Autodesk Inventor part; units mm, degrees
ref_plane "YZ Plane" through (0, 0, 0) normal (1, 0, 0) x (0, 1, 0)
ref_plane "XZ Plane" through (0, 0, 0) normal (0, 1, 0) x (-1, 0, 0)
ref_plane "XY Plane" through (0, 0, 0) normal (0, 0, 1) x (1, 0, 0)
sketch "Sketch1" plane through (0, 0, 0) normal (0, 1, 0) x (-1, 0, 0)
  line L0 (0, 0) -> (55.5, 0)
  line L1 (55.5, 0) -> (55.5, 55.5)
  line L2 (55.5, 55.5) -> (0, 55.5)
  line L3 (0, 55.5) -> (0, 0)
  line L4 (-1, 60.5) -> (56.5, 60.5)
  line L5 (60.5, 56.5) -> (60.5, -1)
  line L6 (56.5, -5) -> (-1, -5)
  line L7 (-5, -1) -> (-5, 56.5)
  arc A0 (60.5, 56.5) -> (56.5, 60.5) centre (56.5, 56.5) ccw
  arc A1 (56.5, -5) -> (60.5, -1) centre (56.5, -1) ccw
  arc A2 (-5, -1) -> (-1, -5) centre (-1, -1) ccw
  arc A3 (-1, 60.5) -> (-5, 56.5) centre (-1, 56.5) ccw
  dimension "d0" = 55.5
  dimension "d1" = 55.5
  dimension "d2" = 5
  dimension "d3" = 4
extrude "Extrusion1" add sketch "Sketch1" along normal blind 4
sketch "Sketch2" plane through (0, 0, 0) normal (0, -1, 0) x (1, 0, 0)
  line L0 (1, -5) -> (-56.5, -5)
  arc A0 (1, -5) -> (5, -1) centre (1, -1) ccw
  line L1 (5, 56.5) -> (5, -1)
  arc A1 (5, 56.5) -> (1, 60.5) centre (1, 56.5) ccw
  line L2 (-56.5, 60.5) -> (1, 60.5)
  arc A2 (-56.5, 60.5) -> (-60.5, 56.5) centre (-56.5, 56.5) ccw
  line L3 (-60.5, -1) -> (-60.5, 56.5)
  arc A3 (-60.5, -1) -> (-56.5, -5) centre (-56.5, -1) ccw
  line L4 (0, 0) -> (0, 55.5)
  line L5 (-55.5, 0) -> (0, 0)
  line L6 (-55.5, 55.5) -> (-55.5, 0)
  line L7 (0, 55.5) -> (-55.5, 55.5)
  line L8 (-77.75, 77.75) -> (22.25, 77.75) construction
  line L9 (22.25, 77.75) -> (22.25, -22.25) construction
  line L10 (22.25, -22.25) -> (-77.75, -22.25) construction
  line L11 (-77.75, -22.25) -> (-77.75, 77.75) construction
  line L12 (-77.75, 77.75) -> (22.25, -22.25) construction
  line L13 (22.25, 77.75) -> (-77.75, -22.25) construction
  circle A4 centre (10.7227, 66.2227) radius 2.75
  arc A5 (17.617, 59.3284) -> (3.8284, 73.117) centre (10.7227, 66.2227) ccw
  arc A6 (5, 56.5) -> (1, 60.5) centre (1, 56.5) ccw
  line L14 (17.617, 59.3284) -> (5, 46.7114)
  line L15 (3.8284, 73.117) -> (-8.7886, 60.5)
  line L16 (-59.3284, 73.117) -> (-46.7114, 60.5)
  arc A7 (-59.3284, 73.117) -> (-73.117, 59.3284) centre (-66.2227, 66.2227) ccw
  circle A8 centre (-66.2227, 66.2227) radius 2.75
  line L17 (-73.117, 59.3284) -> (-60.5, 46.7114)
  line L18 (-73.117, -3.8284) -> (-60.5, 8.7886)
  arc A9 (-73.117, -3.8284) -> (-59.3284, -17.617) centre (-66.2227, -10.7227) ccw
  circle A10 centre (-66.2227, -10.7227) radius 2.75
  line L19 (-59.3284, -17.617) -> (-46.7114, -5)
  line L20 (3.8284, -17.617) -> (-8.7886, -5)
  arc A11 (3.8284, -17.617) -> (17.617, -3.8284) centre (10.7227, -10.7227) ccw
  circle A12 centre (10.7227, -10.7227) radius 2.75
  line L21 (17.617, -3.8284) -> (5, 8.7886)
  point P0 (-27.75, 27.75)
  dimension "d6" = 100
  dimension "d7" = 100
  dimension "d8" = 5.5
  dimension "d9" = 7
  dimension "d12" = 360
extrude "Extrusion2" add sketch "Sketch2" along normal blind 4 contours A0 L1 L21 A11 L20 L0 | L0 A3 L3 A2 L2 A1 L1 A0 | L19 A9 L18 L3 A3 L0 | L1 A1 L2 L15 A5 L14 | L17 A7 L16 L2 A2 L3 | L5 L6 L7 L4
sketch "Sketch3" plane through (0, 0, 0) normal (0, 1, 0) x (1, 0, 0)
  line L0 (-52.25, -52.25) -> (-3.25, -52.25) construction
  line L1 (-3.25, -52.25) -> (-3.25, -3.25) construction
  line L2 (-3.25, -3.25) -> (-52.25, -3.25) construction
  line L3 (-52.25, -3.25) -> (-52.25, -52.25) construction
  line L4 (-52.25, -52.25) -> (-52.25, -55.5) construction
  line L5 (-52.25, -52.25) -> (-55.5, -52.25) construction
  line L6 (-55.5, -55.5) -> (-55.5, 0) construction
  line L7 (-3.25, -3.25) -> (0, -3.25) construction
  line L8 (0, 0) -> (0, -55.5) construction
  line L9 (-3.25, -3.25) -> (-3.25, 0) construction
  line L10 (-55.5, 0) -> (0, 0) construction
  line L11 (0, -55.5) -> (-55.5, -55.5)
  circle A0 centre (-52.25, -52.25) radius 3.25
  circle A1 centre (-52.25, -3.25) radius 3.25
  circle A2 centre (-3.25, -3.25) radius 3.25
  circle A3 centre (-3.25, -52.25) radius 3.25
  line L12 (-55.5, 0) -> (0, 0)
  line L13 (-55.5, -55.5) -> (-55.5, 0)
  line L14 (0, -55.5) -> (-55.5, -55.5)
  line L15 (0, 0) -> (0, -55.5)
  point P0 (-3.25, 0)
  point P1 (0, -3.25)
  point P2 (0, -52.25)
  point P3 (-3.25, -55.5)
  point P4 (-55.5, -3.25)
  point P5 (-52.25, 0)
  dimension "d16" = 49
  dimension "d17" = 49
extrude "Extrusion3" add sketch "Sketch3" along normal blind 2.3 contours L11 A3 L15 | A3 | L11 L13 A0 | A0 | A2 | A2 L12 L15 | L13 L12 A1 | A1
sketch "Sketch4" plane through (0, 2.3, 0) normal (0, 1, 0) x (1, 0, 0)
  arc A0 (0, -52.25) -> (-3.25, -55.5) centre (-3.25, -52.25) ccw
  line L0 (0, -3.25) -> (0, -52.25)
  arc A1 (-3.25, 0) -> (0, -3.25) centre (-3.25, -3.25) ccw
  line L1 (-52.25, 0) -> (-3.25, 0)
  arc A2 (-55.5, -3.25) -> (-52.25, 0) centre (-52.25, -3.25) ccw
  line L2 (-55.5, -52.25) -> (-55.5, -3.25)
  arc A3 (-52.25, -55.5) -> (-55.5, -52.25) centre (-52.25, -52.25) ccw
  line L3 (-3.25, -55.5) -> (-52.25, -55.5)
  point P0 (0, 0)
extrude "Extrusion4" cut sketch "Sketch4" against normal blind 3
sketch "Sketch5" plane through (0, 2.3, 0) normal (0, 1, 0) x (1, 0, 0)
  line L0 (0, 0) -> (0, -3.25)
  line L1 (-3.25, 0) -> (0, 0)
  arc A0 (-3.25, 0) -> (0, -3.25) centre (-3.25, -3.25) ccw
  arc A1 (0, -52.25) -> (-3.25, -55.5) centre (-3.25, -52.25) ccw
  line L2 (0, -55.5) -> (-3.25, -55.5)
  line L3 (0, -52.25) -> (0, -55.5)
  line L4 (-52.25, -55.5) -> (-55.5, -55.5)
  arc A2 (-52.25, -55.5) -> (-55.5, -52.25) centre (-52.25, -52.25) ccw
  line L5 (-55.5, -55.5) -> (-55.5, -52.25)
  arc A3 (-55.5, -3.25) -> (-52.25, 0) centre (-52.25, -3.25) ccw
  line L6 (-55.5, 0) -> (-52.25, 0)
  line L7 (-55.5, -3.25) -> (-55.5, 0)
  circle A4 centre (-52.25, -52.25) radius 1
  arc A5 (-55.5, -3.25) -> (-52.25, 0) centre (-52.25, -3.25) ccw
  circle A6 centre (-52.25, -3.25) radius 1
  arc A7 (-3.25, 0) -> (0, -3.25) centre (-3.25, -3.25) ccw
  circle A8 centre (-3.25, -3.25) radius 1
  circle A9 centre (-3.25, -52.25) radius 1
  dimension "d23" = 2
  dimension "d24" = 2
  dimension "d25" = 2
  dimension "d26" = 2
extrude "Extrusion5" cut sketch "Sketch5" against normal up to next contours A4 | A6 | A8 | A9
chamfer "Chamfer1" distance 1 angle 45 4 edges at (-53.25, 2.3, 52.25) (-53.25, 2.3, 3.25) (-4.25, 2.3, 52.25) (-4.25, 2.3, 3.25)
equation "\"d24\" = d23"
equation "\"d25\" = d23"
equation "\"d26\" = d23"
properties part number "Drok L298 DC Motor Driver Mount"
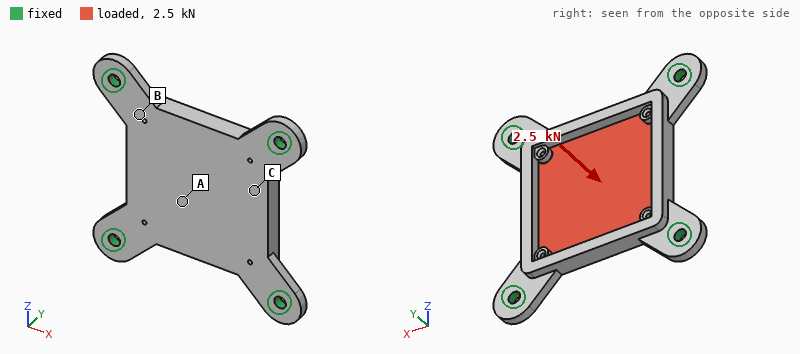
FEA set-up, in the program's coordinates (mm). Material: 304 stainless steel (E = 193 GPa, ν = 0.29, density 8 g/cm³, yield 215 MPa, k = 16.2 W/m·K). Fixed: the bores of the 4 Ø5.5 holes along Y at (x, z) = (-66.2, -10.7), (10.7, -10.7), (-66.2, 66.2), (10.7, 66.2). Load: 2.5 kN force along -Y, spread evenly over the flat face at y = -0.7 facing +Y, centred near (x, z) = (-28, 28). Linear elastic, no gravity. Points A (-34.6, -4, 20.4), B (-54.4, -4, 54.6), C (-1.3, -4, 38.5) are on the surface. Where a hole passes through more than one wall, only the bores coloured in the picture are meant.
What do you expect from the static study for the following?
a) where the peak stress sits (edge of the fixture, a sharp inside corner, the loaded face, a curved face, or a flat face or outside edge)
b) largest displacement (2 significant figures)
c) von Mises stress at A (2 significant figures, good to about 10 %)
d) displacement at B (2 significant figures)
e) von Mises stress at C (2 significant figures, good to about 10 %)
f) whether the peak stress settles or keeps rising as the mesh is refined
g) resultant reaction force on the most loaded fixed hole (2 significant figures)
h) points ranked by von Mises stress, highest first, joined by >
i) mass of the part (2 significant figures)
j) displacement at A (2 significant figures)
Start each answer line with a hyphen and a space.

- edge of the fixture
- 0.11 mm
- 74 MPa
- 0.032 mm
- 41 MPa
- keeps rising
- 770 N
- A > C > B
- 210 g
- 0.10 mm
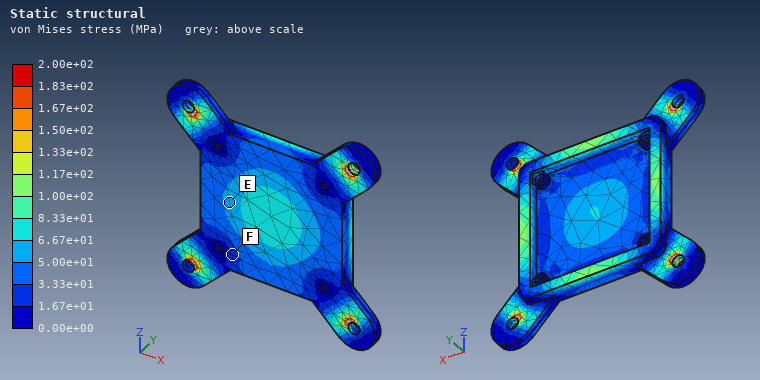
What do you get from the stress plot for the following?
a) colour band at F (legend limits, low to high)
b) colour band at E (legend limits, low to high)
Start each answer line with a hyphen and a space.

- 1.67e+01 to 3.33e+01 MPa
- 5.00e+01 to 6.67e+01 MPa
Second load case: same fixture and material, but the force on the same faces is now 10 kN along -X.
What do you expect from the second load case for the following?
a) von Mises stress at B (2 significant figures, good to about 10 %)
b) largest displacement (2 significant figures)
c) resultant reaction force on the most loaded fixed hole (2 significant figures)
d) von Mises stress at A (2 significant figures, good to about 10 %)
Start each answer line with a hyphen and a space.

- 31 MPa
- 14 µm
- 3.0 kN
- 11 MPa
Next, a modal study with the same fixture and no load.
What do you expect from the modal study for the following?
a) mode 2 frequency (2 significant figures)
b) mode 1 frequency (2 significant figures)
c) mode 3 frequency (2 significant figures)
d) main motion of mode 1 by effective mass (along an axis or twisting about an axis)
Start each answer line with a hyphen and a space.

- 5000 Hz
- 2700 Hz
- 5000 Hz
- along Y
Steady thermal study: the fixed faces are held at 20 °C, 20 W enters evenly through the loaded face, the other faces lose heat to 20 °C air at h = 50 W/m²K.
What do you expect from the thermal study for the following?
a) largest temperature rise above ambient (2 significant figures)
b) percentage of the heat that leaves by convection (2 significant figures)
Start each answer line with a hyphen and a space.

- 50 K
- 70 %
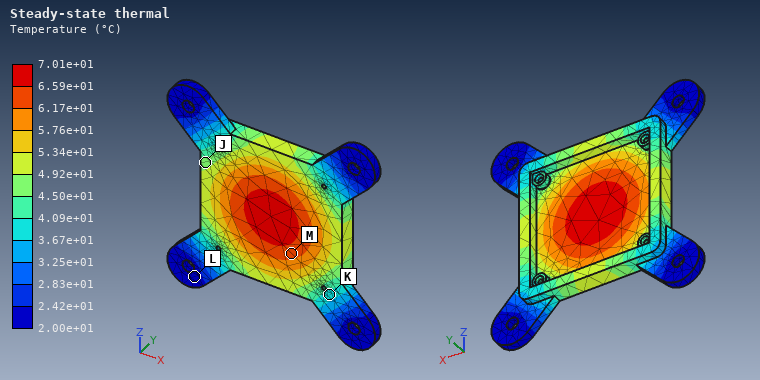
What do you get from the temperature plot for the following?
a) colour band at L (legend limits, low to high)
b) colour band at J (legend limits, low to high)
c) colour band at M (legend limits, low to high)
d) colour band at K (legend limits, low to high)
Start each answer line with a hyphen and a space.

- 2.00e+01 to 2.42e+01 °C
- 4.50e+01 to 4.92e+01 °C
- 6.17e+01 to 6.59e+01 °C
- 3.67e+01 to 4.09e+01 °C
